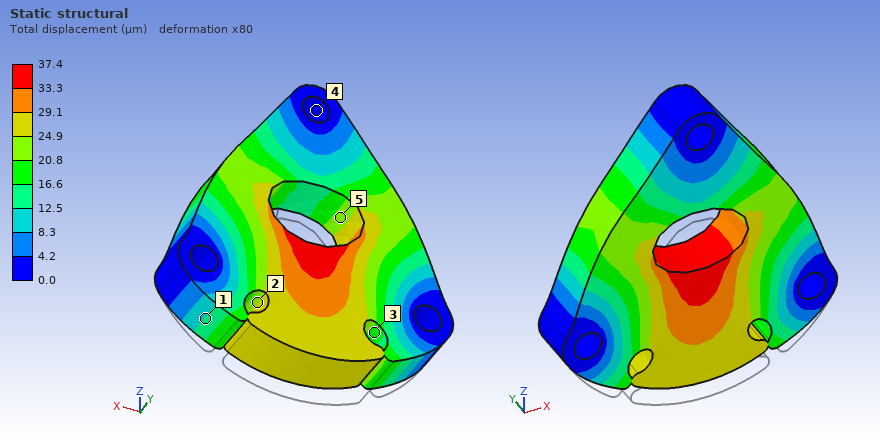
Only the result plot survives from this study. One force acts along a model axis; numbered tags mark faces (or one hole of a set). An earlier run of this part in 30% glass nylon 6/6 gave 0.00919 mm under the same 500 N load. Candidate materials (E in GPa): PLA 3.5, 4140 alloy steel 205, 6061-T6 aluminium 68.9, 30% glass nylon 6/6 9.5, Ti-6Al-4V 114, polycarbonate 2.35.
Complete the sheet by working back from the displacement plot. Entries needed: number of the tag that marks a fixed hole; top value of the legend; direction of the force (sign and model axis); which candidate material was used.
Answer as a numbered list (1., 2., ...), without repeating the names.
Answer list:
1. 4
2. 37.4 µm
3. +Z
4. polycarbonate
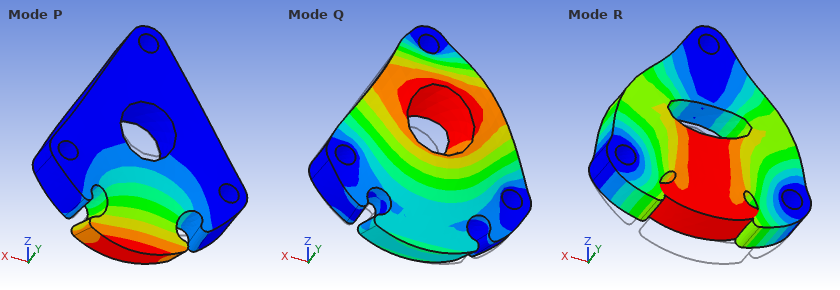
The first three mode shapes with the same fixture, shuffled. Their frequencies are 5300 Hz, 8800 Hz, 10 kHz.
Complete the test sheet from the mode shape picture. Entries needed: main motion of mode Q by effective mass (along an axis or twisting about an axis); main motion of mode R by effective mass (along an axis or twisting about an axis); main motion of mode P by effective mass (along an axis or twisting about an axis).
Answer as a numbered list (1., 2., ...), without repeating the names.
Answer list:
1. along Y
2. along Z
3. along Y
